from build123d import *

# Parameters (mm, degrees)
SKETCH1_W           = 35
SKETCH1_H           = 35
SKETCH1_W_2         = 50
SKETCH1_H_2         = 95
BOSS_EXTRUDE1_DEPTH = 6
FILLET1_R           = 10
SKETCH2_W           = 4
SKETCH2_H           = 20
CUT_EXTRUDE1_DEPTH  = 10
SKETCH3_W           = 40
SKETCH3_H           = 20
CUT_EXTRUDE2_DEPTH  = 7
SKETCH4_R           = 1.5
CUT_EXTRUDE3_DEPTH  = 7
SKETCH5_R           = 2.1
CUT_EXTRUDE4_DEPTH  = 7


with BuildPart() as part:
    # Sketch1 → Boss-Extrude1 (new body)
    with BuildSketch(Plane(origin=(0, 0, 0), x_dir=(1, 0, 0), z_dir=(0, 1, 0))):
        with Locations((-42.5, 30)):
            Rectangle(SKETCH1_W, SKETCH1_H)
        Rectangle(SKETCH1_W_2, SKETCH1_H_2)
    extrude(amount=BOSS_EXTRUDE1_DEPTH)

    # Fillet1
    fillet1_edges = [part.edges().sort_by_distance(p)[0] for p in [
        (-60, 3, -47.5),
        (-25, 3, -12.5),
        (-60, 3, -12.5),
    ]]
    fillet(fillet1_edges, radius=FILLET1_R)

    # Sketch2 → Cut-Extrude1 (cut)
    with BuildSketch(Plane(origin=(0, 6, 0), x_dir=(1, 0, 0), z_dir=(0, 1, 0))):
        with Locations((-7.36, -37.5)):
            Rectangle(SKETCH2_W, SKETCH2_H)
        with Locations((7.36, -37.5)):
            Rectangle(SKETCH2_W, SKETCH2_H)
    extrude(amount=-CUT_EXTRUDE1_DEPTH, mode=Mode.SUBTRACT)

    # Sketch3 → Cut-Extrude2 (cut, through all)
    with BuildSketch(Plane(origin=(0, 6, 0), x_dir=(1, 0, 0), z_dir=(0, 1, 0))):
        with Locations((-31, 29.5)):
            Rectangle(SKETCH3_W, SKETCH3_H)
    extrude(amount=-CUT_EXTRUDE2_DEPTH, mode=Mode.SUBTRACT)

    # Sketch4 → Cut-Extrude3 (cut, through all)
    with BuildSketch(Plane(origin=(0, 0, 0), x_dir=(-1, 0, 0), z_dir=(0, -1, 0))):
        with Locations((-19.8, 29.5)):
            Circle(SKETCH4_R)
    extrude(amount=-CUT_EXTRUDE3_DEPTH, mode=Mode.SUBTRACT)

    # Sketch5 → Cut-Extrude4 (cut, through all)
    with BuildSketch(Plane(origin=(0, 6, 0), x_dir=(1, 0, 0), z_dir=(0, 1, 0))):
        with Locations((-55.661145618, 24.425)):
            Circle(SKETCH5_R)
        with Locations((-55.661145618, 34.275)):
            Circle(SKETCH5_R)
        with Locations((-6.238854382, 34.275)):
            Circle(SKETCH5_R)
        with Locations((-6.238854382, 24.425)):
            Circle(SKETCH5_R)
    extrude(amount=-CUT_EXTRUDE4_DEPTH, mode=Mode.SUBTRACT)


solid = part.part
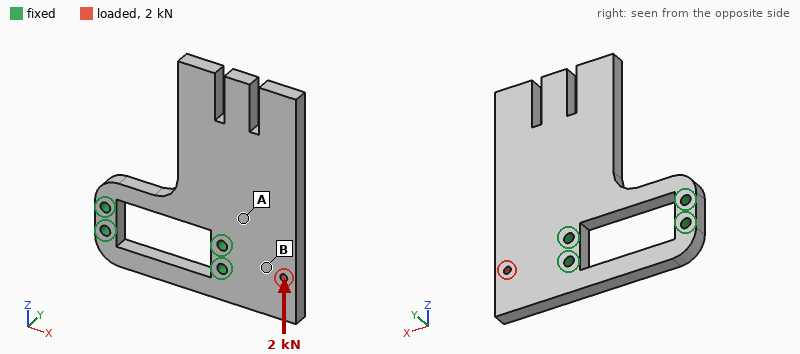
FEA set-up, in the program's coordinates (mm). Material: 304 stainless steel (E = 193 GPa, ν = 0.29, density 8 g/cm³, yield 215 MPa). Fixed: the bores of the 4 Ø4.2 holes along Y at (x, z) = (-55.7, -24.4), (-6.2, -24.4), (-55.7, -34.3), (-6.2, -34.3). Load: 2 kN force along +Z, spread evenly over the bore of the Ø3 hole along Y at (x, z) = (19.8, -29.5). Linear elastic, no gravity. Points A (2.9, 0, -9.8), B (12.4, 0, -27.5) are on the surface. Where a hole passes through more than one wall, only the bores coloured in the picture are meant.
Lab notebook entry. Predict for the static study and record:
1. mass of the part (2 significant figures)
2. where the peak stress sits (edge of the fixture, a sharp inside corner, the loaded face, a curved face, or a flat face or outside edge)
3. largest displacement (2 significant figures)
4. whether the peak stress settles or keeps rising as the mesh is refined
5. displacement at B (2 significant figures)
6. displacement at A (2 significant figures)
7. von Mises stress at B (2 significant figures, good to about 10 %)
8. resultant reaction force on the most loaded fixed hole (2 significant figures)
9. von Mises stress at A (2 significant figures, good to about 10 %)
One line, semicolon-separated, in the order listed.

240 g; edge of the fixture; 26 µm; keeps rising; 7.0 µm; 6.3 µm; 21 MPa; 2.4 kN; 8.0 MPa
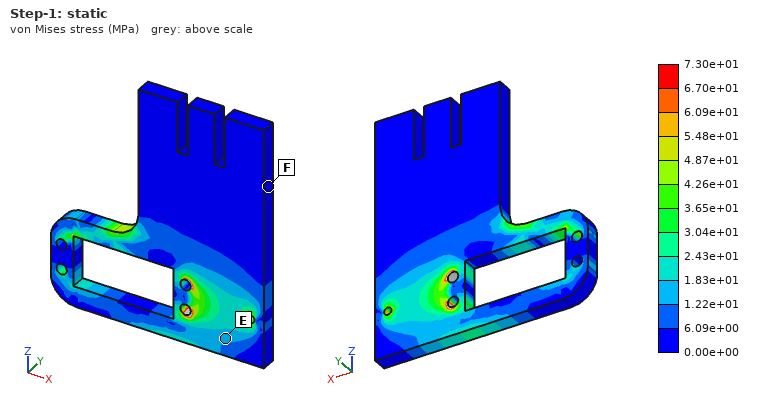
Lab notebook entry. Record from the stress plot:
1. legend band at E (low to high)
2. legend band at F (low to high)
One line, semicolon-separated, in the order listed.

1.22e+01 to 1.83e+01 MPa; 0.00e+00 to 6.09e+00 MPa
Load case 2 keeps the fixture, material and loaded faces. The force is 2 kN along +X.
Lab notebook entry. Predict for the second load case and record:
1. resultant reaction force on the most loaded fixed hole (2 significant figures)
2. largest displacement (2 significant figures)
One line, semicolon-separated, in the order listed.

950 N; 3.1 µm
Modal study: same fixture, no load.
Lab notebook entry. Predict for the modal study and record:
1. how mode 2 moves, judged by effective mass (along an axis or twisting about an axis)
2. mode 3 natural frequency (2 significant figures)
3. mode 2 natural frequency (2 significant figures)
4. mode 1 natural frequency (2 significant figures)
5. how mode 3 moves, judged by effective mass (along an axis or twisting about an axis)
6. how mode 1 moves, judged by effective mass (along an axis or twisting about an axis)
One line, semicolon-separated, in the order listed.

twisting about Z; 2900 Hz; 2100 Hz; 820 Hz; along X; along Y
